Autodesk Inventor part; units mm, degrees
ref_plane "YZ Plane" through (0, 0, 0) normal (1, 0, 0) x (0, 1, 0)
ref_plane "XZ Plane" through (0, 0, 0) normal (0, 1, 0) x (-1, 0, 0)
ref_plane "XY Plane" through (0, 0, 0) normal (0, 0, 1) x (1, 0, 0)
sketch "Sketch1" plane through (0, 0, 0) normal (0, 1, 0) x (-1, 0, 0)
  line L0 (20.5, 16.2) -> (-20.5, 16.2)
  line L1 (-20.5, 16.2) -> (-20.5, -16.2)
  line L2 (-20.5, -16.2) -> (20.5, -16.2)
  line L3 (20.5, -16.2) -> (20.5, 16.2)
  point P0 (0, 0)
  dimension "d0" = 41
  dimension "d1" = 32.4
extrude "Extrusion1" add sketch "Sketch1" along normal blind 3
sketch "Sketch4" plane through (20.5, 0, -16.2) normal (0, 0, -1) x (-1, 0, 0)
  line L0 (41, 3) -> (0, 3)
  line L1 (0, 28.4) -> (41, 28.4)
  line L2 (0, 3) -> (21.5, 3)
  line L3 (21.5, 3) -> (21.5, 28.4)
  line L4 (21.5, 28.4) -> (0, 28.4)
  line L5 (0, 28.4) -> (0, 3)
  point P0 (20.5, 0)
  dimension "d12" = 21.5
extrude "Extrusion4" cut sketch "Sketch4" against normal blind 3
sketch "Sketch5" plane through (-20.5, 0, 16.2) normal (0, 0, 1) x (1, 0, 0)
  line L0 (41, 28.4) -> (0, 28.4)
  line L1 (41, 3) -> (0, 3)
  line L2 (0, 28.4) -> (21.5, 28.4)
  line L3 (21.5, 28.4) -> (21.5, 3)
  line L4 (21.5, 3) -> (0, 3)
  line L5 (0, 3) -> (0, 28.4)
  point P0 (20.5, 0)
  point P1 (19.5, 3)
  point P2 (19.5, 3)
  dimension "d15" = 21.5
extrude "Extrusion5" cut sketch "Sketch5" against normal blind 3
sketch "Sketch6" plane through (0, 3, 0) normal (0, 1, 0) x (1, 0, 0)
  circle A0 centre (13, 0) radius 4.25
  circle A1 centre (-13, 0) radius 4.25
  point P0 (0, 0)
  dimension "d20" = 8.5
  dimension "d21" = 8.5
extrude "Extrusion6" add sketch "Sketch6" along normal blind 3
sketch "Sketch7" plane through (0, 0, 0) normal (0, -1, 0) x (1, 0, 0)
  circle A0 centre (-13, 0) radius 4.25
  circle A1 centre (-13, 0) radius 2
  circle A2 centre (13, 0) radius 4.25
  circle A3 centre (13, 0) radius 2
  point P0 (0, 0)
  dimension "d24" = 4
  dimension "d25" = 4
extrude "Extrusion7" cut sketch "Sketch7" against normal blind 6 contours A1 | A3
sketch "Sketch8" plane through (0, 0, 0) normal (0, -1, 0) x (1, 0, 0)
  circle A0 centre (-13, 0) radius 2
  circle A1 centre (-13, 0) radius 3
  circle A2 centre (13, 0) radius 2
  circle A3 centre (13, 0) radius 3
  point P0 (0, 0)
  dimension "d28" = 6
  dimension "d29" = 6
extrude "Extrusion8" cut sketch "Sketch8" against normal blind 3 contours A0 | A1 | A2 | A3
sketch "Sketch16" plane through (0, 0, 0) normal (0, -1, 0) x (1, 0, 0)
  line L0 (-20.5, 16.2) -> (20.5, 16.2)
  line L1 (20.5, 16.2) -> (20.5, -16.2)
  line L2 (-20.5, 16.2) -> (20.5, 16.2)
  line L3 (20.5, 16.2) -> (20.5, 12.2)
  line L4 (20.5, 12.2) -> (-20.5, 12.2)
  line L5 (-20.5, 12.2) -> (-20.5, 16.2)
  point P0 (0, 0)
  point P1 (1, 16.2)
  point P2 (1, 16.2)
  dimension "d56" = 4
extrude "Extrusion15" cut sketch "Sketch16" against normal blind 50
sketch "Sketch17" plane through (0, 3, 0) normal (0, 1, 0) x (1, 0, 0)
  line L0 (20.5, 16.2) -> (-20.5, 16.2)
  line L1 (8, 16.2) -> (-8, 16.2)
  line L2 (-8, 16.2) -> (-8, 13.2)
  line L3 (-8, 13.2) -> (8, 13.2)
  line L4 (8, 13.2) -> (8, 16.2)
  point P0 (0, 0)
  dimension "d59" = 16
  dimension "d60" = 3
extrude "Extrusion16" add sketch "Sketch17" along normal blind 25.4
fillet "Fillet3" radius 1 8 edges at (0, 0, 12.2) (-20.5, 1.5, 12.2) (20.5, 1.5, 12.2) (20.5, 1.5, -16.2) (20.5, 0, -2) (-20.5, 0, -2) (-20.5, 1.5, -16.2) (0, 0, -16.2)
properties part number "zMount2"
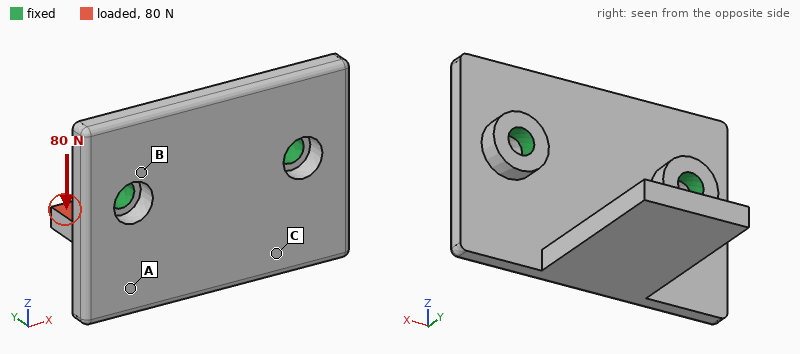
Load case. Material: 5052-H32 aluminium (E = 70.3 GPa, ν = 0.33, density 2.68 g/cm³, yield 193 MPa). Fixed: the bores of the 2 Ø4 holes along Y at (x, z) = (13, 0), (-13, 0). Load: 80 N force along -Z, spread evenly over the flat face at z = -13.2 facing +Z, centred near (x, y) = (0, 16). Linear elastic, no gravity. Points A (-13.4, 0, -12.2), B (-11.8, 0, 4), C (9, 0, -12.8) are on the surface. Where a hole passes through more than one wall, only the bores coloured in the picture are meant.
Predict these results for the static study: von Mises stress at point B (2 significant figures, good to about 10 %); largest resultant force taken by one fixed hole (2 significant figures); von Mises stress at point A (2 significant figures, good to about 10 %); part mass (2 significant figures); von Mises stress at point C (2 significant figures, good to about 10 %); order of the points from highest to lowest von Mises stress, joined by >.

5.2 MPa
41 N
14 MPa
13 g
22 MPa
C > A > B
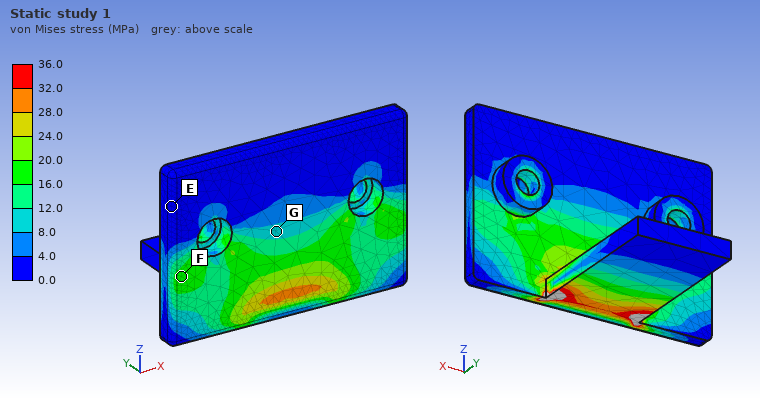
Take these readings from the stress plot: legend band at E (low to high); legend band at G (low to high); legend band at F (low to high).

0.0 to 4.0 MPa
8.0 to 12.0 MPa
16.0 to 20.0 MPa
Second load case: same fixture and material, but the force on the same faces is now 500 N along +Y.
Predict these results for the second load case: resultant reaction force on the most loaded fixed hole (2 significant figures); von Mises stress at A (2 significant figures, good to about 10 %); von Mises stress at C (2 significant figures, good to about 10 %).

310 N
30 MPa
31 MPa
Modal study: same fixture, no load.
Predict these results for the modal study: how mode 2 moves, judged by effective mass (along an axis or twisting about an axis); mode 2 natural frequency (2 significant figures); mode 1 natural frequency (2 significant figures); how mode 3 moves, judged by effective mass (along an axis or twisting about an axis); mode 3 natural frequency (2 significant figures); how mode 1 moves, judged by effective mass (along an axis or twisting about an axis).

along X
4700 Hz
2300 Hz
along Y
6000 Hz
along Z
